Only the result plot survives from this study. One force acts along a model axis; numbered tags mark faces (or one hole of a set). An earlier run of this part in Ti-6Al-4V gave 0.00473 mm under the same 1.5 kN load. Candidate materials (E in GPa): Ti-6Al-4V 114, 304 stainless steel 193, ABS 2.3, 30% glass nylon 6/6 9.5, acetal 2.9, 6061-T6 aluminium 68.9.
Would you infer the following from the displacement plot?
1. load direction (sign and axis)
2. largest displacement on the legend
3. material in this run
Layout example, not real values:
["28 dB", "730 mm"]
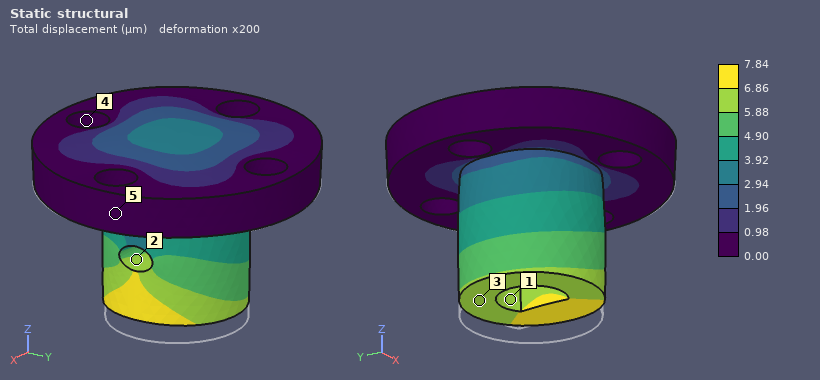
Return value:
["+Z", "7.84 µm", "6061-T6 aluminium"]
